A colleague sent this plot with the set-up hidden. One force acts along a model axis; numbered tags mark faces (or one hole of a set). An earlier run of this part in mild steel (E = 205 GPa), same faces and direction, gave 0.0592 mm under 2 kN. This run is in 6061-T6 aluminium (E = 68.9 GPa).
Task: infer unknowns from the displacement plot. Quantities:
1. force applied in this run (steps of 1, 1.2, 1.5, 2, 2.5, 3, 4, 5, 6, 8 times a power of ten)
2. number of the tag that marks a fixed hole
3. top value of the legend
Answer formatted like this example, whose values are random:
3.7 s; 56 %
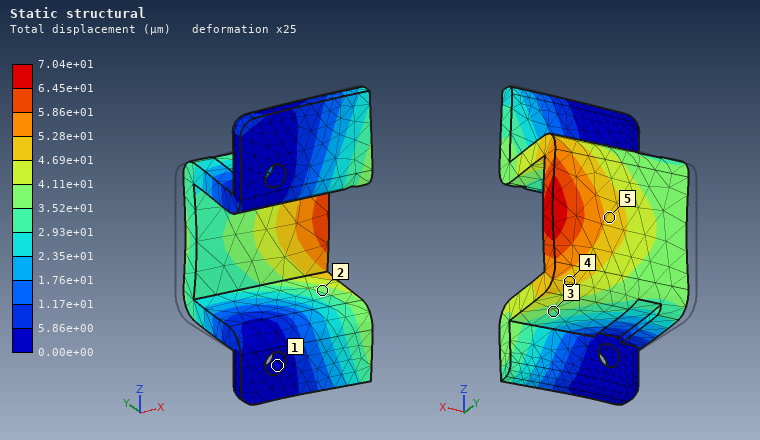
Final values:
800 N; 1; 7.04e+01 µm
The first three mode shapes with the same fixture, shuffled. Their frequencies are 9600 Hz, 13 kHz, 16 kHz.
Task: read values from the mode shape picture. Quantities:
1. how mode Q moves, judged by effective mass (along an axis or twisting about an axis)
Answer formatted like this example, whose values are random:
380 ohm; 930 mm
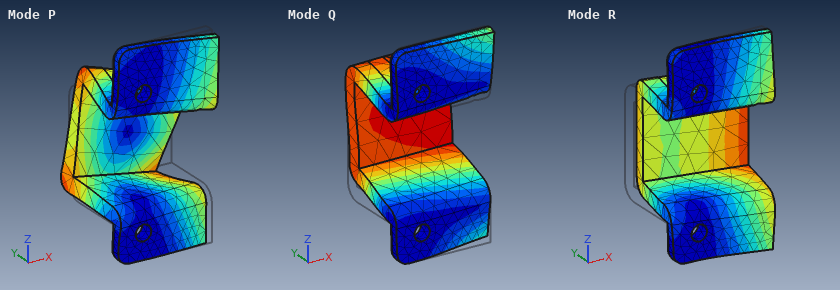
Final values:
along Z
